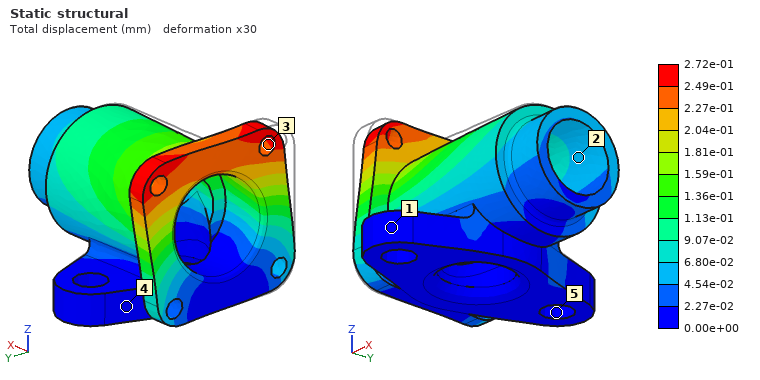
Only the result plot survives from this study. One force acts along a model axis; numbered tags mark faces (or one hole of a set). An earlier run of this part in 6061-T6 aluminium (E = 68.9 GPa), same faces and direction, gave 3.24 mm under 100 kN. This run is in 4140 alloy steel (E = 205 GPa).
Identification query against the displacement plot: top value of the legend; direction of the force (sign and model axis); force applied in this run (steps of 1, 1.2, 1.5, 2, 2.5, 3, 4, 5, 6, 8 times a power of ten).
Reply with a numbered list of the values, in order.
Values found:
1. 2.72e-01 mm
2. +Y
3. 25 kN
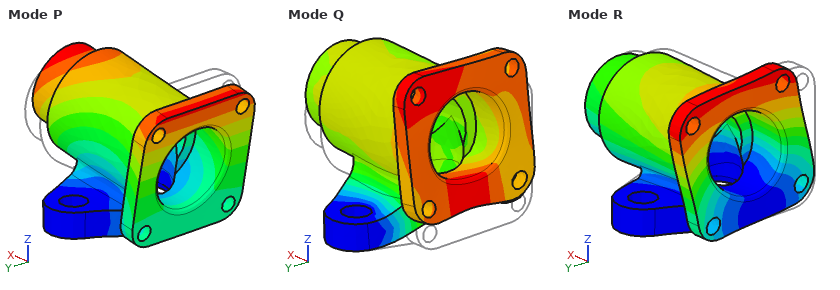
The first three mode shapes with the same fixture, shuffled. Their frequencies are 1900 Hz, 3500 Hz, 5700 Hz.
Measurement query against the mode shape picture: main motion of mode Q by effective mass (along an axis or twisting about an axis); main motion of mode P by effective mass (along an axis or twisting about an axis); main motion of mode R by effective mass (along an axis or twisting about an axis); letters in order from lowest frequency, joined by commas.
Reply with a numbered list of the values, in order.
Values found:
1. along Z
2. along X
3. along Y
4. P, R, Q
